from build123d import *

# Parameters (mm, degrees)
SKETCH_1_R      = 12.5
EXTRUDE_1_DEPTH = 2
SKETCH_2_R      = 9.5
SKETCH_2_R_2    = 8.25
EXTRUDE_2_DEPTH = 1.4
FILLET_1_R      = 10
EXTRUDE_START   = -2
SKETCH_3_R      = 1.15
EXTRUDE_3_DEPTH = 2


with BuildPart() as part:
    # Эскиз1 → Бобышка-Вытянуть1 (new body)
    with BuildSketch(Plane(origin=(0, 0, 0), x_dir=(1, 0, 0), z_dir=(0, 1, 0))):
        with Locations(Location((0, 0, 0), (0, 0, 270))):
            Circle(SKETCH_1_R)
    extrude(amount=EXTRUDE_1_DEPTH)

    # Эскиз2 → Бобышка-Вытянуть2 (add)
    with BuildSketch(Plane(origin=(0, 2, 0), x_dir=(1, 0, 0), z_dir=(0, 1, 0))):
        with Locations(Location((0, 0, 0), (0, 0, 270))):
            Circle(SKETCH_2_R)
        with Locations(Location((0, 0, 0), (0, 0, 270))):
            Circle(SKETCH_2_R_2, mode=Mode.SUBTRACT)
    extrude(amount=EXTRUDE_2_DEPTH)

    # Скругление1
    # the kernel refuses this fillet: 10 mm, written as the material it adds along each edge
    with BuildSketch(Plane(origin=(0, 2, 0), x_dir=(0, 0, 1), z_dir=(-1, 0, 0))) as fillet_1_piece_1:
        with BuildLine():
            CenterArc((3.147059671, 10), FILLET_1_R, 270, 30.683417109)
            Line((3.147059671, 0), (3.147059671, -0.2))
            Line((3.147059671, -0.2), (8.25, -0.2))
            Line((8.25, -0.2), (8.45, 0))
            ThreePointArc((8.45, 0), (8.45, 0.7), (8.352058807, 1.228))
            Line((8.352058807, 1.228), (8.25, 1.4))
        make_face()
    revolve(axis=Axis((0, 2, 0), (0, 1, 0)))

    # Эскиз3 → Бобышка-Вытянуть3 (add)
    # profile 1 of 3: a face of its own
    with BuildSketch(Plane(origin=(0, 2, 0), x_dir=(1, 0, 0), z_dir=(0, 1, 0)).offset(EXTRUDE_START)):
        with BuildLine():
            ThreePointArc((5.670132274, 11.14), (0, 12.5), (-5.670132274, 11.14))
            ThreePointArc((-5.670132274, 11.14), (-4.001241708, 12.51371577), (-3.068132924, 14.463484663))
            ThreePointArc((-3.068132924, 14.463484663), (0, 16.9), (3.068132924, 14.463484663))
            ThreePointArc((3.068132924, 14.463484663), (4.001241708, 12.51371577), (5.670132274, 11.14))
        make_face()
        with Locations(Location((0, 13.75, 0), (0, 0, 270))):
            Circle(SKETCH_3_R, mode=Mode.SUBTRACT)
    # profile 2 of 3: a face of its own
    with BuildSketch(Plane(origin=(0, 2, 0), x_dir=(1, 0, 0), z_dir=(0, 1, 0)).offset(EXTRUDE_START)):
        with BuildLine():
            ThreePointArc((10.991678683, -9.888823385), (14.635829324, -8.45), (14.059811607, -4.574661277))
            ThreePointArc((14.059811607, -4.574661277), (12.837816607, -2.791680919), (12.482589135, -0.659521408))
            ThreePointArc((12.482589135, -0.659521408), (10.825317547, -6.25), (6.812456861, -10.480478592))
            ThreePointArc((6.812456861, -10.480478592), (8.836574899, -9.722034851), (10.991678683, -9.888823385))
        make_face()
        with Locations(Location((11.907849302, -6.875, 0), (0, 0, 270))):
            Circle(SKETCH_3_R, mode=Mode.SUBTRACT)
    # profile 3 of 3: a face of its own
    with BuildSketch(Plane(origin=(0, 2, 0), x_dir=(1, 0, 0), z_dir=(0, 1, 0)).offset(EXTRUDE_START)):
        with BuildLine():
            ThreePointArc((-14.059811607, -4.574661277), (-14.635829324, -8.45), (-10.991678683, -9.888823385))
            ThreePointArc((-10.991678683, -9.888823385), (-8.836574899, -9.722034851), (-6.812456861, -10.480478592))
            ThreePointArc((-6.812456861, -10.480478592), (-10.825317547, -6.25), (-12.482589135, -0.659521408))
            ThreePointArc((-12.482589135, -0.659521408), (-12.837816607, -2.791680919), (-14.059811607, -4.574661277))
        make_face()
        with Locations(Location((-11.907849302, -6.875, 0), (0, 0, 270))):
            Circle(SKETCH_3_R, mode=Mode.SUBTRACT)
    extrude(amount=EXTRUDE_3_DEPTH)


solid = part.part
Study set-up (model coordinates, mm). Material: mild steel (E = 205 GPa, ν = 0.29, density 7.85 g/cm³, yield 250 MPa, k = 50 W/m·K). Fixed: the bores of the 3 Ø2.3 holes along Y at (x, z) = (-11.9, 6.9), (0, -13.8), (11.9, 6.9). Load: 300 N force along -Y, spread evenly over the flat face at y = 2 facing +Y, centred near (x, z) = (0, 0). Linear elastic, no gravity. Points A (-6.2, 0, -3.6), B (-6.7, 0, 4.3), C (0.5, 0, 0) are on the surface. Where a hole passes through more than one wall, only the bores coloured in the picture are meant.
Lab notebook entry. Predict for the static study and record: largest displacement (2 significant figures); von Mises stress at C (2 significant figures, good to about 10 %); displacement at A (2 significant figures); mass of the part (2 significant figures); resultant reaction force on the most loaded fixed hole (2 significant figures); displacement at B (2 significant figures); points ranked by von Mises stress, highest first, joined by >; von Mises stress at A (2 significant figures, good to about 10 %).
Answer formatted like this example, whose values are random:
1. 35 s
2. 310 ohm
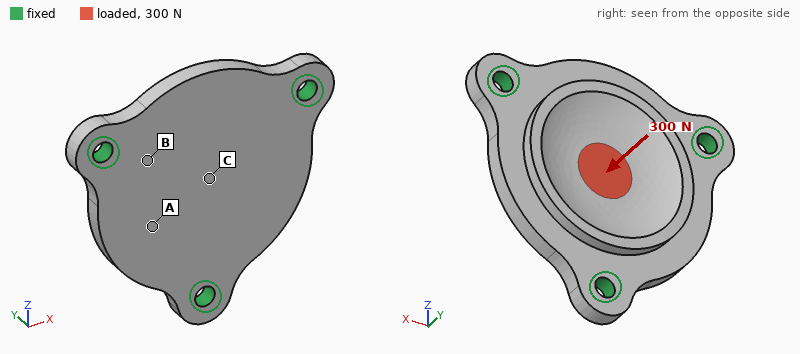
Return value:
1. 7.9 µm
2. 63 MPa
3. 4.5 µm
4. 10 g
5. 110 N
6. 3.3 µm
7. C > A > B
8. 27 MPa
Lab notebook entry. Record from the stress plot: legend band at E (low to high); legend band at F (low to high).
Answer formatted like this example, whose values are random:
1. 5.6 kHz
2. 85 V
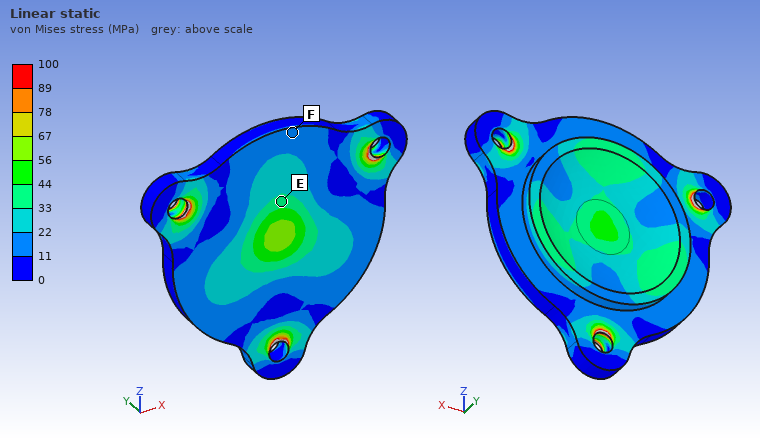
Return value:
1. 33 to 44 MPa
2. 11 to 22 MPa
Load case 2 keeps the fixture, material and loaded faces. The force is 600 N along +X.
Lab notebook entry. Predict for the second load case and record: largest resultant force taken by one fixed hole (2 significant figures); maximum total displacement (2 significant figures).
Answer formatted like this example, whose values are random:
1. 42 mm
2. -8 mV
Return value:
1. 250 N
2. 1.7 µm
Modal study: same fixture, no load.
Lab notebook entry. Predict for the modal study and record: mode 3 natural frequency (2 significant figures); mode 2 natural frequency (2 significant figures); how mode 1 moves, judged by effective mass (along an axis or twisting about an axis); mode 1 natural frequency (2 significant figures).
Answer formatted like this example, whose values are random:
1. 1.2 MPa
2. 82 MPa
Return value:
1. 20 kHz
2. 20 kHz
3. along Y
4. 17 kHz
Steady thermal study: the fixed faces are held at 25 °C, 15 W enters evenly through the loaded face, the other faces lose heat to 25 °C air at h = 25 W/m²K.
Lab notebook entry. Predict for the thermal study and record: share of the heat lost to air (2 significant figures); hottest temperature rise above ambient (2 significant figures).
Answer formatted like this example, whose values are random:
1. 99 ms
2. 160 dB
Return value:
1. 5.9 %
2. 68 K
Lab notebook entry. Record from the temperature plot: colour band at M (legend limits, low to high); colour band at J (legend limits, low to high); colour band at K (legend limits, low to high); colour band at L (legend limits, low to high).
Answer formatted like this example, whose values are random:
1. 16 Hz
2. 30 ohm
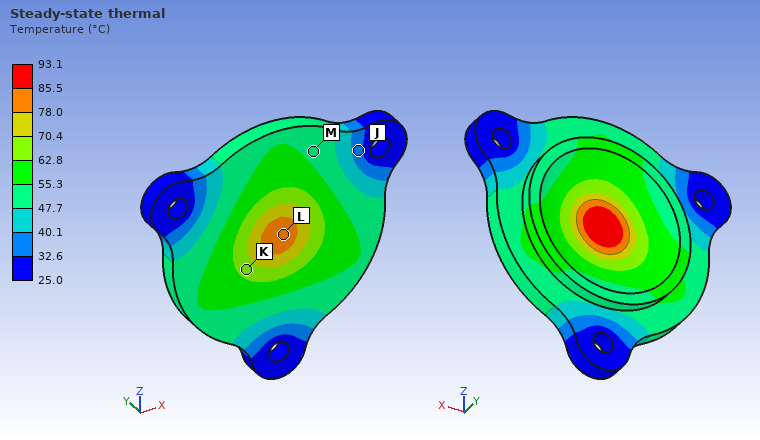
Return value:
1. 47.7 to 55.3 °C
2. 32.6 to 40.1 °C
3. 62.8 to 70.4 °C
4. 78.0 to 85.5 °C
